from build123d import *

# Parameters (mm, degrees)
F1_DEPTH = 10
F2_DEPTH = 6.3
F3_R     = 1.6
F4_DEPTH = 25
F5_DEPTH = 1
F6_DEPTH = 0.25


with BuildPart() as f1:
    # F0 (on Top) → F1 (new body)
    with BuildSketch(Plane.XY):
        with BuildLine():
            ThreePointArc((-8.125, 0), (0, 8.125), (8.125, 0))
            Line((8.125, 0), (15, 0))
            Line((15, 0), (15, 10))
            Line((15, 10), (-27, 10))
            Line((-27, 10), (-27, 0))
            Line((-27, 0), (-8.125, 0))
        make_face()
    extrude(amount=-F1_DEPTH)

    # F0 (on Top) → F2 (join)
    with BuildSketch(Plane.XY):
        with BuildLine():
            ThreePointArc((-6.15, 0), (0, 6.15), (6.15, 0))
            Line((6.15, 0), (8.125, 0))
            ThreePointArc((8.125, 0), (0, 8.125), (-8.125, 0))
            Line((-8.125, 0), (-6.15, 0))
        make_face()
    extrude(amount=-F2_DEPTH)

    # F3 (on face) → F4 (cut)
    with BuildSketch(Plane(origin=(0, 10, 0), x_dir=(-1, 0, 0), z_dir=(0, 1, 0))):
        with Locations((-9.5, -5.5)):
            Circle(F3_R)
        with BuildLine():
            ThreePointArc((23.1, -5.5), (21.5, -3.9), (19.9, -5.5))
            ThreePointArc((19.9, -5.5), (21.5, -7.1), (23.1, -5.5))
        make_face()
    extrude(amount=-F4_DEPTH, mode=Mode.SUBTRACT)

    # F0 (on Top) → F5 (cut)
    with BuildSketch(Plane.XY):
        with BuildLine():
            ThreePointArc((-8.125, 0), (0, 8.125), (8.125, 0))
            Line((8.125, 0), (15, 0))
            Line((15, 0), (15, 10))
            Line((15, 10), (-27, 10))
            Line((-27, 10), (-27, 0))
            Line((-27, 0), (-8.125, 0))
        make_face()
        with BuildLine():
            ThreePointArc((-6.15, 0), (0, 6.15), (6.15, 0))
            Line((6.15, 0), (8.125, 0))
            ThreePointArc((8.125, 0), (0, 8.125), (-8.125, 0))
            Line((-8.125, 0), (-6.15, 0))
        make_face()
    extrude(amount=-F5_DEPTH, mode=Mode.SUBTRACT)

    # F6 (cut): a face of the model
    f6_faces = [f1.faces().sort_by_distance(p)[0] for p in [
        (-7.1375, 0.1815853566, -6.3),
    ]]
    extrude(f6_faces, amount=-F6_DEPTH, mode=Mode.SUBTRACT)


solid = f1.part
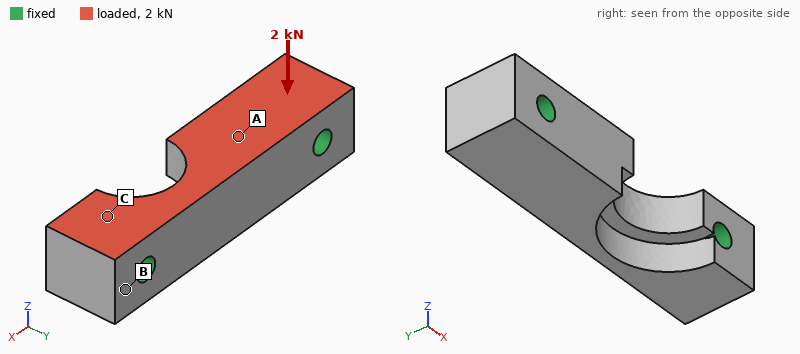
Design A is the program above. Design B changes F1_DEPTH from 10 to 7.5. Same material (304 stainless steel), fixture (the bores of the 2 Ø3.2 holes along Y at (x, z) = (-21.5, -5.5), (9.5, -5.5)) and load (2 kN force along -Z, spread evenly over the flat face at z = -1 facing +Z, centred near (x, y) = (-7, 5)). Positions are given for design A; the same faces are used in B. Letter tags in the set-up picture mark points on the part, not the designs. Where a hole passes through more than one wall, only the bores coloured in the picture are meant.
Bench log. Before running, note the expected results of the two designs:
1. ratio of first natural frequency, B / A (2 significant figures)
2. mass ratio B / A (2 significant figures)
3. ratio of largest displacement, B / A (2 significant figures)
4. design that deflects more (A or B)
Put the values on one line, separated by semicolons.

0.93; 0.73; 1.6; B
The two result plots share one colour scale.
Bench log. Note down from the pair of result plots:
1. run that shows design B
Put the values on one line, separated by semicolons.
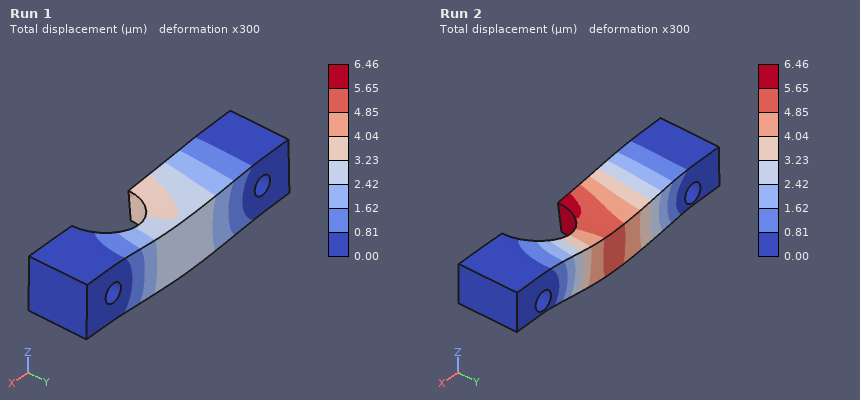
Run 2
